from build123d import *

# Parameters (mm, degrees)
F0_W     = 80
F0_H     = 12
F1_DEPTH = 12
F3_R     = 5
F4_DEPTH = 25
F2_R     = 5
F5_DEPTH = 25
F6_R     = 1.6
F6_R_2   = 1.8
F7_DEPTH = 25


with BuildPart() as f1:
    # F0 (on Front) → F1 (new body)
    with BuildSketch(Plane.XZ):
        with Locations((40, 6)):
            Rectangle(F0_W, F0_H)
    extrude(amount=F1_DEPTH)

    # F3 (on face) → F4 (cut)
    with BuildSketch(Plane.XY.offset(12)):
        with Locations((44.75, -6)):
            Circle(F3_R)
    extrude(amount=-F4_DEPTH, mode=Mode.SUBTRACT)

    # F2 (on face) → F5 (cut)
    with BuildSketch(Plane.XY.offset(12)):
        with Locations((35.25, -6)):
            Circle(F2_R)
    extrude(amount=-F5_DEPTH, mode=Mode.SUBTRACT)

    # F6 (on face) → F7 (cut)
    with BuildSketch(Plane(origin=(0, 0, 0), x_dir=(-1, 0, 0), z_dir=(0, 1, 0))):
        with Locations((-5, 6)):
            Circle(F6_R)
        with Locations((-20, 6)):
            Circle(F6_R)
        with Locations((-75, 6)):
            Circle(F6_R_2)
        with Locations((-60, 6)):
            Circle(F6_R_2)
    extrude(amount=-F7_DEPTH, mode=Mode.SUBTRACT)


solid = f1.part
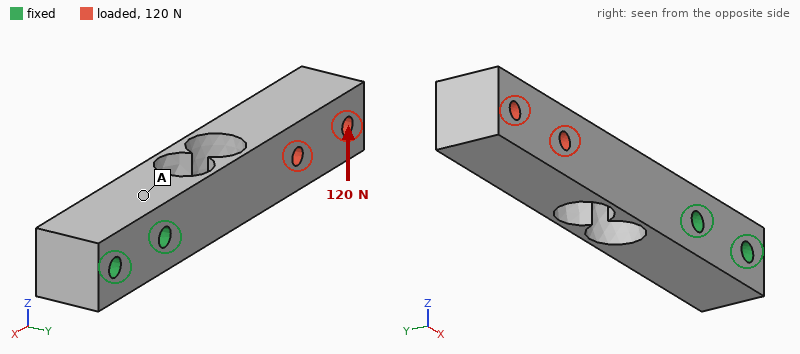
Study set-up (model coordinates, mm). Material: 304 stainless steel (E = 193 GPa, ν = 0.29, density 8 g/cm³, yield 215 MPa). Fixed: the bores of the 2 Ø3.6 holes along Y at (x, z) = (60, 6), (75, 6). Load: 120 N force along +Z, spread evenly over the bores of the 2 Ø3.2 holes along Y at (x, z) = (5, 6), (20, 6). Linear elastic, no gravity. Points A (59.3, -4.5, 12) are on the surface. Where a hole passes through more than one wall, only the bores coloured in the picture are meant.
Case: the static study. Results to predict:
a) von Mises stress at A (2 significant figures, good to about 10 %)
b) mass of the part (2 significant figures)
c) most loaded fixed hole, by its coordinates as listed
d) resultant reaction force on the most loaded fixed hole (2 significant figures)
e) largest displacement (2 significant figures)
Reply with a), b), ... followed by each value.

a) 15 MPa
b) 74 g
c) (60, 6)
d) 320 N
e) 58 µm
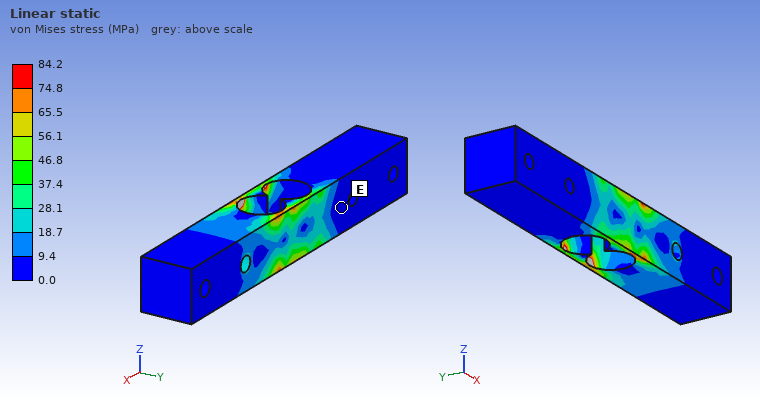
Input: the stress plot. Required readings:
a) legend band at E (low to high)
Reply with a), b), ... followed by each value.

a) 0.0 to 9.4 MPa
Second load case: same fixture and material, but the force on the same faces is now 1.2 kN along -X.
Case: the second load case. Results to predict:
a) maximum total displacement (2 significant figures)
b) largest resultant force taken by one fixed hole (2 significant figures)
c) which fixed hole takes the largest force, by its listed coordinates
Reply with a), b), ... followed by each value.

a) 6.3 µm
b) 1.1 kN
c) (60, 6)
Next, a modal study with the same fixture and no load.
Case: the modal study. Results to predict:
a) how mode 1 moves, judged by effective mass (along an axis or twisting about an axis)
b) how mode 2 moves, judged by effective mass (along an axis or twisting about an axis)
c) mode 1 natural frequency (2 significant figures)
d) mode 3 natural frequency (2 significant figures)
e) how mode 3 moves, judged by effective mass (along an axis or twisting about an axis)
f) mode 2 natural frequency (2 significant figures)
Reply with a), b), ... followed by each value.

a) along Y
b) along Z
c) 1100 Hz
d) 5900 Hz
e) twisting about X
f) 1500 Hz
